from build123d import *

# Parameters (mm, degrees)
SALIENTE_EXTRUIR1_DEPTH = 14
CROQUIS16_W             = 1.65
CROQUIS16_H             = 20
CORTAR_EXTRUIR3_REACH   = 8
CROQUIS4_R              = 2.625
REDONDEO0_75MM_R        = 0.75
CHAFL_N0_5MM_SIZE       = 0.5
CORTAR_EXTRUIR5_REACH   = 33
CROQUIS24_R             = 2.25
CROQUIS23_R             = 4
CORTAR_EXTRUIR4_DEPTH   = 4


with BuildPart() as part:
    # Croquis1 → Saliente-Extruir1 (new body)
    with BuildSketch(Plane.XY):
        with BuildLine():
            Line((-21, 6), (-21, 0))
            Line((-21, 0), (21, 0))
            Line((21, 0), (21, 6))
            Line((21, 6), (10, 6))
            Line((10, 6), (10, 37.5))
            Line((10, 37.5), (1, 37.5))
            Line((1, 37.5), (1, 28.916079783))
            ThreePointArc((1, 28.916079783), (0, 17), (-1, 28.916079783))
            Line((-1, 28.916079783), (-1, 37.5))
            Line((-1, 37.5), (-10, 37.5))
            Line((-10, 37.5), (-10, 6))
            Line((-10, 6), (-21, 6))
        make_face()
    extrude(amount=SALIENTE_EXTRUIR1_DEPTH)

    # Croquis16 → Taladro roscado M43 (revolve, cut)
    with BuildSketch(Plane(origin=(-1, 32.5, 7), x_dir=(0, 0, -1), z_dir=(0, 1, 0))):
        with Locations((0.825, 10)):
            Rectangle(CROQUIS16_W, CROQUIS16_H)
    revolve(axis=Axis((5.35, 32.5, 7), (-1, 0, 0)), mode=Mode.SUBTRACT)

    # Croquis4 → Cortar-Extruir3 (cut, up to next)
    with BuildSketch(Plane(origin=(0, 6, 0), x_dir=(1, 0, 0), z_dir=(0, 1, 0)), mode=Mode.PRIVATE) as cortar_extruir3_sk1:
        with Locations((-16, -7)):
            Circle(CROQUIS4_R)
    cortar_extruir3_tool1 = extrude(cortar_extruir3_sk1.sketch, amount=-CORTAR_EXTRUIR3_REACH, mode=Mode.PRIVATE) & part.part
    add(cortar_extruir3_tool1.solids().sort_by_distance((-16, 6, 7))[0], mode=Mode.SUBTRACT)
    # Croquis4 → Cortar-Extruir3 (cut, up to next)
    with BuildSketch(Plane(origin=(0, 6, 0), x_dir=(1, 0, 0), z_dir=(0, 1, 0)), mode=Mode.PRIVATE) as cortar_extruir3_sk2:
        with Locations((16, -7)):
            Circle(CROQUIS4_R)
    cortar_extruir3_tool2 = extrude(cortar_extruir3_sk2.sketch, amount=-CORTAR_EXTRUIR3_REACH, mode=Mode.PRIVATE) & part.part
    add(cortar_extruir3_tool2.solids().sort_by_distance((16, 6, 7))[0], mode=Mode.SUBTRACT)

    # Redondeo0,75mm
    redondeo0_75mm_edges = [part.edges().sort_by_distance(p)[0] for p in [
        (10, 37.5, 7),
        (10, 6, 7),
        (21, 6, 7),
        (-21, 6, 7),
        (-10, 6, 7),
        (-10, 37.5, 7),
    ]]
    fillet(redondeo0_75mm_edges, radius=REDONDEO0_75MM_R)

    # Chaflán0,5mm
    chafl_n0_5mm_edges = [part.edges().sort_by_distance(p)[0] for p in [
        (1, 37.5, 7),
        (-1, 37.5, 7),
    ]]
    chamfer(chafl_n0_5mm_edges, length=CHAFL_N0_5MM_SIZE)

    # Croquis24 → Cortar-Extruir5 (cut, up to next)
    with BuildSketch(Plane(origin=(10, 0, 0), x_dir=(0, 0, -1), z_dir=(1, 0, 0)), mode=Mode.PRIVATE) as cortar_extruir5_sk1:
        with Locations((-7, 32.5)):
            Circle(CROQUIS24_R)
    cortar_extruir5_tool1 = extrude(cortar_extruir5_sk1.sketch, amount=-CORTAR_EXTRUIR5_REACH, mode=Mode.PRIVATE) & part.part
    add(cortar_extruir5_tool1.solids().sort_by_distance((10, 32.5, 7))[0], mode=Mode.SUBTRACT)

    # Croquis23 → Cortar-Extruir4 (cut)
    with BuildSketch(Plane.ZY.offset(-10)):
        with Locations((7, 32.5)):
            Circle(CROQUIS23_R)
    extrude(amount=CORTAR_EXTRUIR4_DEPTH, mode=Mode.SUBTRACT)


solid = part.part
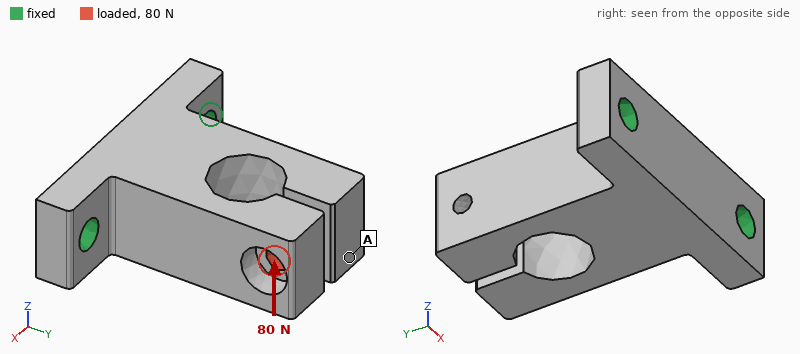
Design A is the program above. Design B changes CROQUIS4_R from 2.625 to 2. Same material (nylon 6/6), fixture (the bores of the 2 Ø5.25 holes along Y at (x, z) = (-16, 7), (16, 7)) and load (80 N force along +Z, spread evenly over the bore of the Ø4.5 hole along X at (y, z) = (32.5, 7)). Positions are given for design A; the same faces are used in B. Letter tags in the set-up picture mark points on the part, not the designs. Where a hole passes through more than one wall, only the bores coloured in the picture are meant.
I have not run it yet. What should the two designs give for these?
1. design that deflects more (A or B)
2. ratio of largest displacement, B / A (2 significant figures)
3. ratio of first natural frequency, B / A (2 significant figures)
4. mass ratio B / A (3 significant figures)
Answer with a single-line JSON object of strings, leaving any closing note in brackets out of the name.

{"design that deflects more": "B", "ratio of largest displacement, B / A": "1.1", "ratio of first natural frequency, B / A": "0.93", "mass ratio B / A": "1.01"}
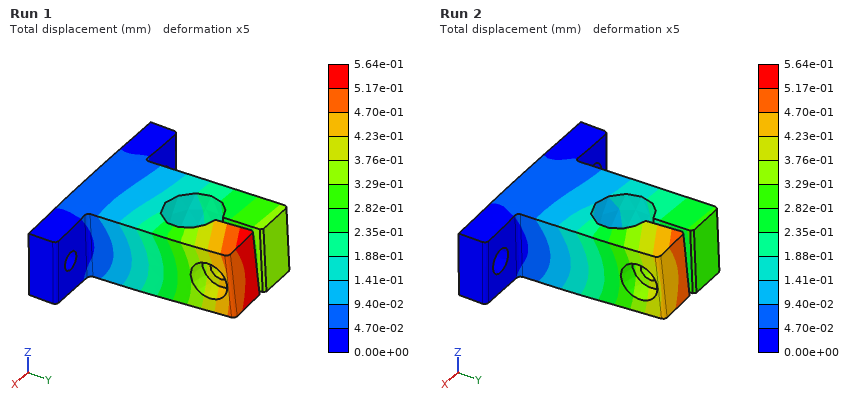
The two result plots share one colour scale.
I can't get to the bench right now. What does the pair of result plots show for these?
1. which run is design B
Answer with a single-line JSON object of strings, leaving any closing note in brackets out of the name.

{"which run is design B": "Run 1"}
